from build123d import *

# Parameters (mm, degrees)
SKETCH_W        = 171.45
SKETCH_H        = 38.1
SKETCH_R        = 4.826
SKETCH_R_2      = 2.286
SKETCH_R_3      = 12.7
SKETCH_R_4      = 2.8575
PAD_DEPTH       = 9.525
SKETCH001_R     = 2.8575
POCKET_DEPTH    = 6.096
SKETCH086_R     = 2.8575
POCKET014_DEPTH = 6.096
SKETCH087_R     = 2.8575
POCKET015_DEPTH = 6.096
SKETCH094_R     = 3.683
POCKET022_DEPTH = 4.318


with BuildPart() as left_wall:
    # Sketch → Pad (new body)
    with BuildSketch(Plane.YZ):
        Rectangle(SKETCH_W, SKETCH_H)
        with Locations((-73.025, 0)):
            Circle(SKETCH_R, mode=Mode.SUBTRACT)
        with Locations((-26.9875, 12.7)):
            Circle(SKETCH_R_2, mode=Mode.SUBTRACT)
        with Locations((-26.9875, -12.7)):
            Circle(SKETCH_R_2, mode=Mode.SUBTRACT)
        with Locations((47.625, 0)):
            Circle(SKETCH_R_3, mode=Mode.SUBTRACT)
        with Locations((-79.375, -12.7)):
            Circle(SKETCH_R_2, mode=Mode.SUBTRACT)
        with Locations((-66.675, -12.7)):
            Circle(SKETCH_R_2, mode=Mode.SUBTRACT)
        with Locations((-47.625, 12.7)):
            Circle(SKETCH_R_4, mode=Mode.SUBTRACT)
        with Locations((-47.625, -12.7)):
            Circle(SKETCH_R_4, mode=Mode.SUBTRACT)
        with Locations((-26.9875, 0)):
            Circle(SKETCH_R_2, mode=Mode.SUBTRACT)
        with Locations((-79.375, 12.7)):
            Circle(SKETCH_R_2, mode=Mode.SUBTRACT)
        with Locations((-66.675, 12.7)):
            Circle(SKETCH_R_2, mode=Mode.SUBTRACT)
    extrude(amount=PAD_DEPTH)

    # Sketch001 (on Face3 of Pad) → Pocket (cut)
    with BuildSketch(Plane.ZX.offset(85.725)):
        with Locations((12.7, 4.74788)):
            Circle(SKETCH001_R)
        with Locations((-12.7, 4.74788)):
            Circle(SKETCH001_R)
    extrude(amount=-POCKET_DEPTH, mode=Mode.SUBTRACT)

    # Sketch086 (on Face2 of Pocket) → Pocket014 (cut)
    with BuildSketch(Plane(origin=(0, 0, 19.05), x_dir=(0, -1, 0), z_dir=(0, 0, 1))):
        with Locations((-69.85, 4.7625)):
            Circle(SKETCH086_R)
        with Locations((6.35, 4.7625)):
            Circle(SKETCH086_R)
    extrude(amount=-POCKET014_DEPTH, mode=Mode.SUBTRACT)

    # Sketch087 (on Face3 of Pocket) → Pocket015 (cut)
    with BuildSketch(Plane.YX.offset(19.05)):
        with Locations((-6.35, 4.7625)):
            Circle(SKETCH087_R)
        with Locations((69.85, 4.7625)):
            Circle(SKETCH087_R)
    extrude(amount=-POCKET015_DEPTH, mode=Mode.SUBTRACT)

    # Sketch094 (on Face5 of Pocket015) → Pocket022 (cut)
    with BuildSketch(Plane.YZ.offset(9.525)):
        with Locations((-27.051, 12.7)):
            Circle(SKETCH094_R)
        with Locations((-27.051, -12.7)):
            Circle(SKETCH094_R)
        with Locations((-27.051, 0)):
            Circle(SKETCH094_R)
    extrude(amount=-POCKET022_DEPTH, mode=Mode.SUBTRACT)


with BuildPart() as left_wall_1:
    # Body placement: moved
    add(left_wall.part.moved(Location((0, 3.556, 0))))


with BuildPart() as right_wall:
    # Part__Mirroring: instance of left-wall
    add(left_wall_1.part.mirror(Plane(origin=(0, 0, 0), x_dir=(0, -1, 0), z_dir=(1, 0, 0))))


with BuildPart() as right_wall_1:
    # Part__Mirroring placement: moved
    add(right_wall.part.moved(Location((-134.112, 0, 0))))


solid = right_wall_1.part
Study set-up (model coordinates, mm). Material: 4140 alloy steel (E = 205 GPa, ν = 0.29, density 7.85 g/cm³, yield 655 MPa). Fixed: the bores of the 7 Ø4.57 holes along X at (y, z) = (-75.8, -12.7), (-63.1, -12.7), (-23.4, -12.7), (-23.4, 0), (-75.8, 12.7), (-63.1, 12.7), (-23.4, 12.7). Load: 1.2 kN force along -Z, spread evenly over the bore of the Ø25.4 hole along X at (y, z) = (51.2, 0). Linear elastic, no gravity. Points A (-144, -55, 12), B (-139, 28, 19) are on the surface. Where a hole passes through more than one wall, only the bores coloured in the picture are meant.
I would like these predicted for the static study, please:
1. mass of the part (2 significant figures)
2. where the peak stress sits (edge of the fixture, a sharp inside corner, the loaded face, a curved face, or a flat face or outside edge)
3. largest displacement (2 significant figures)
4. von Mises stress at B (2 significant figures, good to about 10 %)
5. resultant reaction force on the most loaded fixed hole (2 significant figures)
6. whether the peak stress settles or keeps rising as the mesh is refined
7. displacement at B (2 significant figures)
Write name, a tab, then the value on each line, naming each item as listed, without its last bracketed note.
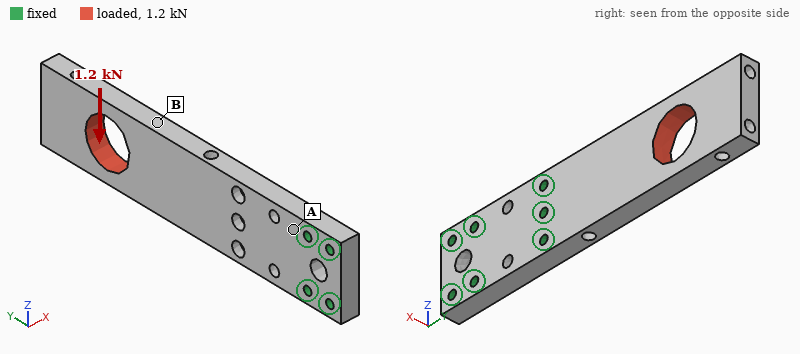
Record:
mass of the part	420 g
where the peak stress sits	edge of the fixture
largest displacement	53 µm
von Mises stress at B	16 MPa
resultant reaction force on the most loaded fixed hole	2.8 kN
whether the peak stress settles or keeps rising as the mesh is refined	keeps rising
displacement at B	18 µm
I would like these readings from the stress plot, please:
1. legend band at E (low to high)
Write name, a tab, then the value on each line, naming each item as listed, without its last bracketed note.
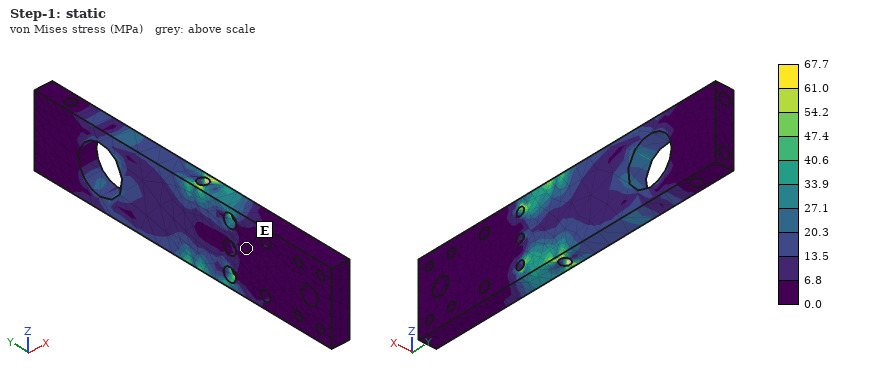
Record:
legend band at E	0.0 to 6.8 MPa
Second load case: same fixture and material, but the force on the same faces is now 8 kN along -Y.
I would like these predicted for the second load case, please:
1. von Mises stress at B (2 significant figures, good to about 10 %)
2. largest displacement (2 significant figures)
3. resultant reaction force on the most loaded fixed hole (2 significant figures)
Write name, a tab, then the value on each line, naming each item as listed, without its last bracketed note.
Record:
von Mises stress at B	34 MPa
largest displacement	31 µm
resultant reaction force on the most loaded fixed hole	2.4 kN
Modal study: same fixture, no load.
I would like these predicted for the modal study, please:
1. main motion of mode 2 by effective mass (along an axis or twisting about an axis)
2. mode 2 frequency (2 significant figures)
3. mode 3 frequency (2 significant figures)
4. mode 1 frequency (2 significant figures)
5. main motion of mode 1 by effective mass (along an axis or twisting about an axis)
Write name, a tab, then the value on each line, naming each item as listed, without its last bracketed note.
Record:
main motion of mode 2 by effective mass	along Z
mode 2 frequency	2100 Hz
mode 3 frequency	3100 Hz
mode 1 frequency	610 Hz
main motion of mode 1 by effective mass	along X
